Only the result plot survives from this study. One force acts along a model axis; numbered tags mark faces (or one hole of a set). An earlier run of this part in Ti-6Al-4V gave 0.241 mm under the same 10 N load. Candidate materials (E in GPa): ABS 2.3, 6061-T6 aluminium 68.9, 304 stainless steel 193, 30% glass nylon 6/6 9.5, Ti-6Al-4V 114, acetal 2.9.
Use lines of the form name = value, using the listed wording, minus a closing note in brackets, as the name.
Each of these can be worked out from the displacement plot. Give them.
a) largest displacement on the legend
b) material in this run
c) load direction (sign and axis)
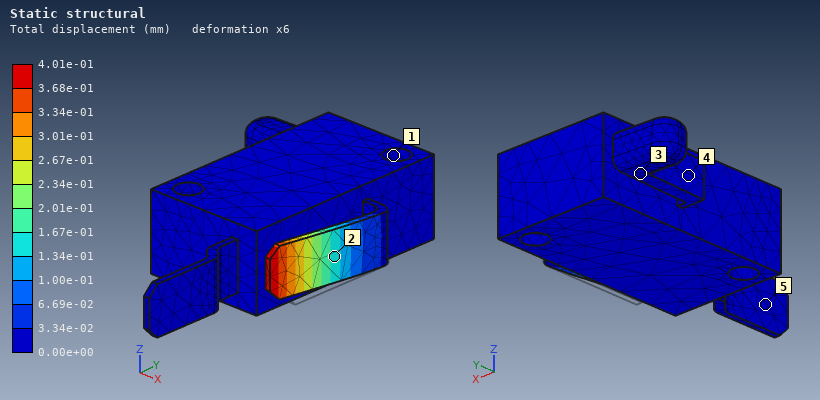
largest displacement on the legend = 4.01e-01 mm
material in this run = 6061-T6 aluminium
load direction = -X
